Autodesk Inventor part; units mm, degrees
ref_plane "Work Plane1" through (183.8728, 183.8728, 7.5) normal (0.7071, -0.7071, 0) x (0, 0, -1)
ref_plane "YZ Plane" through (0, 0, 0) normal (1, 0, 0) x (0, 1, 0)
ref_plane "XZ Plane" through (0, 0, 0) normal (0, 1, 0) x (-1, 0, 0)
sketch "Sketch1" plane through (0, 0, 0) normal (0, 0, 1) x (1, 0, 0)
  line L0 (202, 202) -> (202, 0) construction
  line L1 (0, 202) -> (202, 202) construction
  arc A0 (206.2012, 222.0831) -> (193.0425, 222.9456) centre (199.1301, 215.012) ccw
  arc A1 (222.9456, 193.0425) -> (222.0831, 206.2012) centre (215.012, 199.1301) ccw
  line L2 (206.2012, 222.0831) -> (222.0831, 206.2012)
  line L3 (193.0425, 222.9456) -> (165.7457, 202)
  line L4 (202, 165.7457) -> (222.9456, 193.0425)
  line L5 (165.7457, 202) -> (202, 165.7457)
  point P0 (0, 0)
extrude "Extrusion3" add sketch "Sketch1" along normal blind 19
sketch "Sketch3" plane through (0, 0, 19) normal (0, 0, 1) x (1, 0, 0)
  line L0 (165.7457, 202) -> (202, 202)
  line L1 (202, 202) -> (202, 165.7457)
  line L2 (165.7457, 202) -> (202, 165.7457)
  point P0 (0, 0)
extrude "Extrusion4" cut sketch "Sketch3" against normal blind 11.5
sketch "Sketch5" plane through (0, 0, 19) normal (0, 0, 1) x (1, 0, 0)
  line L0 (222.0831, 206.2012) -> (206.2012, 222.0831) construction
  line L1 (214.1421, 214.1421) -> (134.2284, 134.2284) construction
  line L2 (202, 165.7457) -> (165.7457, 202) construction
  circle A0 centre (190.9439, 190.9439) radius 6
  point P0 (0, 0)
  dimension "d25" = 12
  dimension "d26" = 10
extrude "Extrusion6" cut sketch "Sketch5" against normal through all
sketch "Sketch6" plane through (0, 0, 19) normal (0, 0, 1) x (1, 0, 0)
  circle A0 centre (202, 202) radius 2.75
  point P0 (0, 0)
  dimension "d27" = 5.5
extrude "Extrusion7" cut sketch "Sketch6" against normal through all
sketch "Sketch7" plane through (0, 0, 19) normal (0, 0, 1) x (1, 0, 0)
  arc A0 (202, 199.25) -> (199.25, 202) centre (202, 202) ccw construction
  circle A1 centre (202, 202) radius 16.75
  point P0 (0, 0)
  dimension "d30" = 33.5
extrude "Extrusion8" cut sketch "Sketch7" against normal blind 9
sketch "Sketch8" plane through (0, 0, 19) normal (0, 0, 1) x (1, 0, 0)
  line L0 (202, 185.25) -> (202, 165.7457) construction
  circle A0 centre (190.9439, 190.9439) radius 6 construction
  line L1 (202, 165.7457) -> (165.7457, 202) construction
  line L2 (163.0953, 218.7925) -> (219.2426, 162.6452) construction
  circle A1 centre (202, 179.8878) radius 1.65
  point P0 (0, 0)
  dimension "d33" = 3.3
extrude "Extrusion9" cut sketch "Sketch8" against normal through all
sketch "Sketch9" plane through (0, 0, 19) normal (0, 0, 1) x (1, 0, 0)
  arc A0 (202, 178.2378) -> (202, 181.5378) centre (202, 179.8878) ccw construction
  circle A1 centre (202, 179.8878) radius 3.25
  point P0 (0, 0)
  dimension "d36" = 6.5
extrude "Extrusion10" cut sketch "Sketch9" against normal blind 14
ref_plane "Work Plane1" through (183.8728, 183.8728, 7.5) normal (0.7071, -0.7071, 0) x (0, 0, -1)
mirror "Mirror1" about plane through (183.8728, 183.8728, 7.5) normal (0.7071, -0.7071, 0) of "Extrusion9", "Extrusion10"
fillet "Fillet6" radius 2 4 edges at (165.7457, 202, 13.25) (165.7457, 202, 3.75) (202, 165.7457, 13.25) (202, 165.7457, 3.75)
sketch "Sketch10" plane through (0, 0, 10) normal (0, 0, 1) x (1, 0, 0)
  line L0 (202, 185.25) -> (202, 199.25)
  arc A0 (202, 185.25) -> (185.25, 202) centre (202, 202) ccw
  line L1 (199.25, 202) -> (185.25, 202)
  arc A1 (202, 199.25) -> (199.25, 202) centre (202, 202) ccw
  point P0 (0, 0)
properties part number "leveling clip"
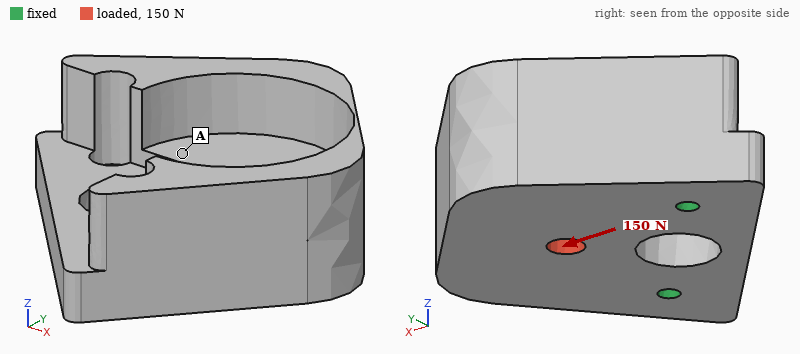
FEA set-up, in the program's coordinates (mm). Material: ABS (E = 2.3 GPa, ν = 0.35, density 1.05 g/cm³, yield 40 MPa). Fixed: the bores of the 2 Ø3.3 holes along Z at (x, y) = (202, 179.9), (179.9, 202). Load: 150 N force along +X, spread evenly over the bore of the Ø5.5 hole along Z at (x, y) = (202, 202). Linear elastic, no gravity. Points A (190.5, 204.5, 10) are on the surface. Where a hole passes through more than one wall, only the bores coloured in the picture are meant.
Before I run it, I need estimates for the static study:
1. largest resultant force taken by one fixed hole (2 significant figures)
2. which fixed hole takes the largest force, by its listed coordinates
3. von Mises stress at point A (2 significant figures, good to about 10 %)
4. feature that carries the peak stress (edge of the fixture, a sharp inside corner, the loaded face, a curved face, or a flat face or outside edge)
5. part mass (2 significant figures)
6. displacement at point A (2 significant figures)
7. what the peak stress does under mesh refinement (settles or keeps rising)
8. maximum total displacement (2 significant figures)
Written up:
120 N
(179.9, 202)
0.58 MPa
edge of the fixture
22 g
15 µm
keeps rising
34 µm
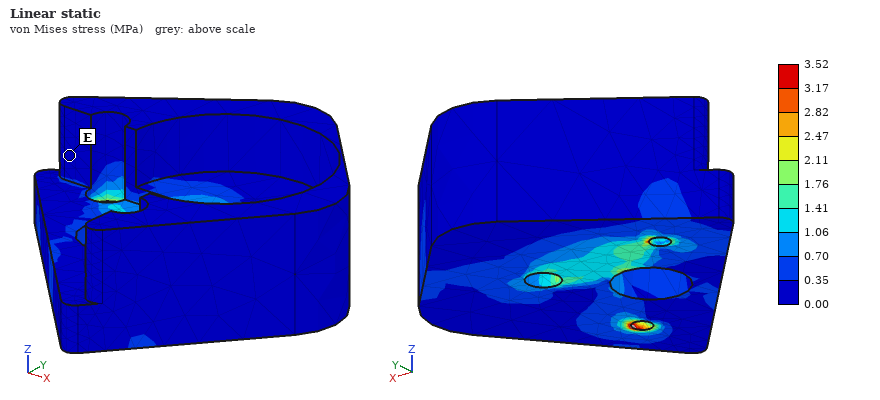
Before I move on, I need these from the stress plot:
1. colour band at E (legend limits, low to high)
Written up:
0.00 to 0.35 MPa
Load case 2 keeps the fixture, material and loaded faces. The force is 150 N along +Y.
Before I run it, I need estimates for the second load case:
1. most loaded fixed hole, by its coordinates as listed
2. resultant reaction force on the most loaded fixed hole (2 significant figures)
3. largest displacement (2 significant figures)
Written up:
(202, 179.9)
120 N
34 µm
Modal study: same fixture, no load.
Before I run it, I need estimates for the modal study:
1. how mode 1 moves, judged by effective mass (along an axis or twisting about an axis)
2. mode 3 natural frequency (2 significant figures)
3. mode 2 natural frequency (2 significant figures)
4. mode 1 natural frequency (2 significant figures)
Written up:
along Z
3300 Hz
2300 Hz
950 Hz
